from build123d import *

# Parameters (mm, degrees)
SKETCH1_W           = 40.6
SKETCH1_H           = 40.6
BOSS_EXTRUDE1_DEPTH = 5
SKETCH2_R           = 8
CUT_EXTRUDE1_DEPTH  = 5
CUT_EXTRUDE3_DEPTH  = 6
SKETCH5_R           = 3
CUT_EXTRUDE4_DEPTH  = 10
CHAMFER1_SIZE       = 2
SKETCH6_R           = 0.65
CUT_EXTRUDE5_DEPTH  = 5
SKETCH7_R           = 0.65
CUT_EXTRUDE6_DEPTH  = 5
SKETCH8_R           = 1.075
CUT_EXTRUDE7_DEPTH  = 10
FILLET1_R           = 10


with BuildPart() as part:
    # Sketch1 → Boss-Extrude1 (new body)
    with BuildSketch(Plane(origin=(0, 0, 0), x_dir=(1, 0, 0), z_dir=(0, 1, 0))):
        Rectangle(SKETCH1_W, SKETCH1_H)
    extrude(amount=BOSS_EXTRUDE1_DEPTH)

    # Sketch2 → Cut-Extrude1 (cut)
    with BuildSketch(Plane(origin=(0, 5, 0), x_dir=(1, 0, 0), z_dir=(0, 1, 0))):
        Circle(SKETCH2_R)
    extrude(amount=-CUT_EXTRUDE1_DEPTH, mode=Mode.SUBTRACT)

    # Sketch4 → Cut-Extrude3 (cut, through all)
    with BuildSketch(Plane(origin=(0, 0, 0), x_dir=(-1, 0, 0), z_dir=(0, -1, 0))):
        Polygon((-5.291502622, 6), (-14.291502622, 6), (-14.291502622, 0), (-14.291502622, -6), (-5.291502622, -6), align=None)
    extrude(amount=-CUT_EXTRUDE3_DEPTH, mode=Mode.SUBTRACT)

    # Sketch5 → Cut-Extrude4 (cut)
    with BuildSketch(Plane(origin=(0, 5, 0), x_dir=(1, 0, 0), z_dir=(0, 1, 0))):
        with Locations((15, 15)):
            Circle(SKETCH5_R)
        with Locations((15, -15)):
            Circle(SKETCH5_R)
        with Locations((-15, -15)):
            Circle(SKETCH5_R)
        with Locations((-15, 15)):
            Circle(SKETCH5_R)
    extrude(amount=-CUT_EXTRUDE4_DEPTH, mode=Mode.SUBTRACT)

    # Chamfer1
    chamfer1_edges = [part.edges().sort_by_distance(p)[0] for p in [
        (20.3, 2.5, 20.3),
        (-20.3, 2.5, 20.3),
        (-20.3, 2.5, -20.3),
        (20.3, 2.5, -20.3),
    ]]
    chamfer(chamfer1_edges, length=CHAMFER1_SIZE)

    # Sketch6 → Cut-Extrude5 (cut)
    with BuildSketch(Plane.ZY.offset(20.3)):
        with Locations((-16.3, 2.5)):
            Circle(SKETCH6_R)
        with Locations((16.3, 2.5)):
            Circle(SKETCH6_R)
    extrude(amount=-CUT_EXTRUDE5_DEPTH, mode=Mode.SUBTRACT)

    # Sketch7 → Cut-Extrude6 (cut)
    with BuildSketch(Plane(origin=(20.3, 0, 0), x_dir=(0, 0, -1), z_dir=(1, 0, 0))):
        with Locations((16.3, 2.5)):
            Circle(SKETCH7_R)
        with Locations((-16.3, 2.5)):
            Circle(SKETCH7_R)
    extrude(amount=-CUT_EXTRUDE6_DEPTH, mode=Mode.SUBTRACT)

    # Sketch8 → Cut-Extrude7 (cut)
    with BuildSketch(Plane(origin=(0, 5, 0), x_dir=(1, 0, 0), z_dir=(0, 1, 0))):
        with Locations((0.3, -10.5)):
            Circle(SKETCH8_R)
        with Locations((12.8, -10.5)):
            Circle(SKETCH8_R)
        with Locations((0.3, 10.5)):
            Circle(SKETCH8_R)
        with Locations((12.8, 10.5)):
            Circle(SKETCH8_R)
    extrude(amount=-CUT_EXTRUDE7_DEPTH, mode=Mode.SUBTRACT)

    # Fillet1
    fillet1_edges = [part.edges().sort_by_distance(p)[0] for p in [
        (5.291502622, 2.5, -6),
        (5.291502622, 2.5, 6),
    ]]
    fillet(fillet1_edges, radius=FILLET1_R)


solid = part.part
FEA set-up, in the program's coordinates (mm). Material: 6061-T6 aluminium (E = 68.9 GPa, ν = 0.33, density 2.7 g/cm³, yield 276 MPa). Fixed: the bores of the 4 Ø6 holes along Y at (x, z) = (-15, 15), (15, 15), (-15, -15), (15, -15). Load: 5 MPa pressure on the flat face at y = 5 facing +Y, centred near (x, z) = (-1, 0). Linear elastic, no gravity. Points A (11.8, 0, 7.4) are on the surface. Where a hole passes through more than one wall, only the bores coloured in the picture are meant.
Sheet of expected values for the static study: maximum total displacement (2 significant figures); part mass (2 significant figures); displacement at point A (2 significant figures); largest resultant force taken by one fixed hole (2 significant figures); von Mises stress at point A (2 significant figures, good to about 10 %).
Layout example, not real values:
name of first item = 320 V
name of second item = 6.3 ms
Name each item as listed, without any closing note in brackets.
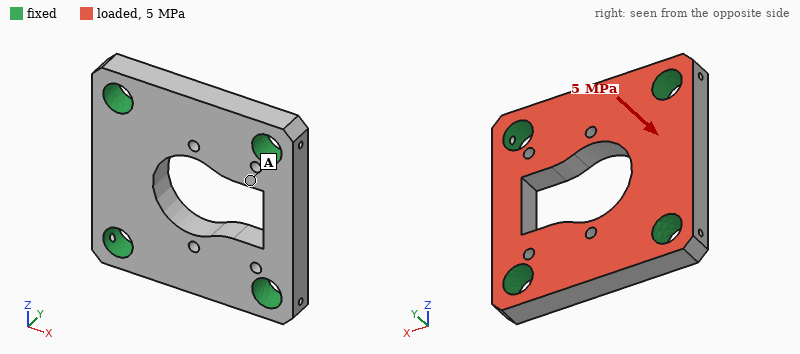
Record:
maximum total displacement = 19 µm
part mass = 16 g
displacement at point A = 8.9 µm
largest resultant force taken by one fixed hole = 1.6 kN
von Mises stress at point A = 19 MPa
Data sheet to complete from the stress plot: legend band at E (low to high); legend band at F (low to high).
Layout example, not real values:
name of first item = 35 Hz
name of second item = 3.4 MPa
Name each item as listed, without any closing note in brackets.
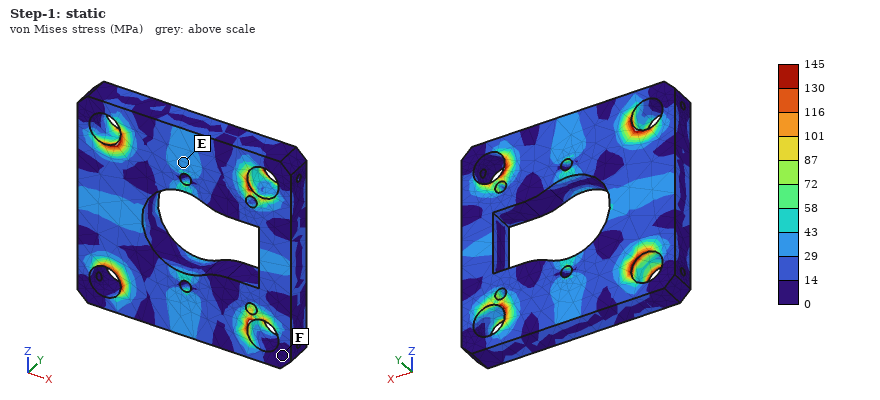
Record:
legend band at E = 29 to 43 MPa
legend band at F = 0 to 14 MPa
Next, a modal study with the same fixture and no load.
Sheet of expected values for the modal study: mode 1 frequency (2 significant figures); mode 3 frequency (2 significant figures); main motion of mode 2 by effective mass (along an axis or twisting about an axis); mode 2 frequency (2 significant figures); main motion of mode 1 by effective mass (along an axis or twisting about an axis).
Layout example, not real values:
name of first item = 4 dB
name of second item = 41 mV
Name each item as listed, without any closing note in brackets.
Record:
mode 1 frequency = 27 kHz
mode 3 frequency = 33 kHz
main motion of mode 2 by effective mass = twisting about X
mode 2 frequency = 31 kHz
main motion of mode 1 by effective mass = along Y
